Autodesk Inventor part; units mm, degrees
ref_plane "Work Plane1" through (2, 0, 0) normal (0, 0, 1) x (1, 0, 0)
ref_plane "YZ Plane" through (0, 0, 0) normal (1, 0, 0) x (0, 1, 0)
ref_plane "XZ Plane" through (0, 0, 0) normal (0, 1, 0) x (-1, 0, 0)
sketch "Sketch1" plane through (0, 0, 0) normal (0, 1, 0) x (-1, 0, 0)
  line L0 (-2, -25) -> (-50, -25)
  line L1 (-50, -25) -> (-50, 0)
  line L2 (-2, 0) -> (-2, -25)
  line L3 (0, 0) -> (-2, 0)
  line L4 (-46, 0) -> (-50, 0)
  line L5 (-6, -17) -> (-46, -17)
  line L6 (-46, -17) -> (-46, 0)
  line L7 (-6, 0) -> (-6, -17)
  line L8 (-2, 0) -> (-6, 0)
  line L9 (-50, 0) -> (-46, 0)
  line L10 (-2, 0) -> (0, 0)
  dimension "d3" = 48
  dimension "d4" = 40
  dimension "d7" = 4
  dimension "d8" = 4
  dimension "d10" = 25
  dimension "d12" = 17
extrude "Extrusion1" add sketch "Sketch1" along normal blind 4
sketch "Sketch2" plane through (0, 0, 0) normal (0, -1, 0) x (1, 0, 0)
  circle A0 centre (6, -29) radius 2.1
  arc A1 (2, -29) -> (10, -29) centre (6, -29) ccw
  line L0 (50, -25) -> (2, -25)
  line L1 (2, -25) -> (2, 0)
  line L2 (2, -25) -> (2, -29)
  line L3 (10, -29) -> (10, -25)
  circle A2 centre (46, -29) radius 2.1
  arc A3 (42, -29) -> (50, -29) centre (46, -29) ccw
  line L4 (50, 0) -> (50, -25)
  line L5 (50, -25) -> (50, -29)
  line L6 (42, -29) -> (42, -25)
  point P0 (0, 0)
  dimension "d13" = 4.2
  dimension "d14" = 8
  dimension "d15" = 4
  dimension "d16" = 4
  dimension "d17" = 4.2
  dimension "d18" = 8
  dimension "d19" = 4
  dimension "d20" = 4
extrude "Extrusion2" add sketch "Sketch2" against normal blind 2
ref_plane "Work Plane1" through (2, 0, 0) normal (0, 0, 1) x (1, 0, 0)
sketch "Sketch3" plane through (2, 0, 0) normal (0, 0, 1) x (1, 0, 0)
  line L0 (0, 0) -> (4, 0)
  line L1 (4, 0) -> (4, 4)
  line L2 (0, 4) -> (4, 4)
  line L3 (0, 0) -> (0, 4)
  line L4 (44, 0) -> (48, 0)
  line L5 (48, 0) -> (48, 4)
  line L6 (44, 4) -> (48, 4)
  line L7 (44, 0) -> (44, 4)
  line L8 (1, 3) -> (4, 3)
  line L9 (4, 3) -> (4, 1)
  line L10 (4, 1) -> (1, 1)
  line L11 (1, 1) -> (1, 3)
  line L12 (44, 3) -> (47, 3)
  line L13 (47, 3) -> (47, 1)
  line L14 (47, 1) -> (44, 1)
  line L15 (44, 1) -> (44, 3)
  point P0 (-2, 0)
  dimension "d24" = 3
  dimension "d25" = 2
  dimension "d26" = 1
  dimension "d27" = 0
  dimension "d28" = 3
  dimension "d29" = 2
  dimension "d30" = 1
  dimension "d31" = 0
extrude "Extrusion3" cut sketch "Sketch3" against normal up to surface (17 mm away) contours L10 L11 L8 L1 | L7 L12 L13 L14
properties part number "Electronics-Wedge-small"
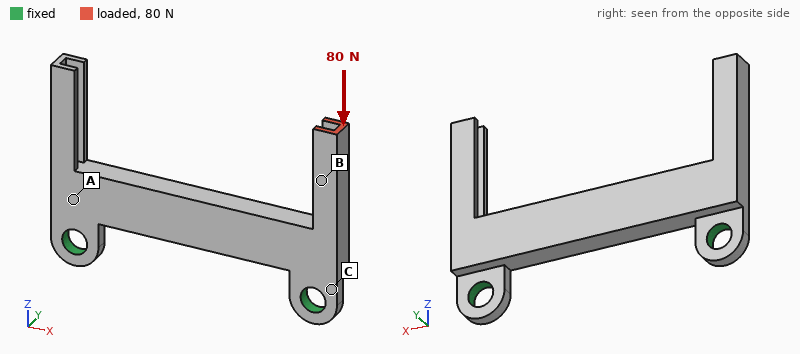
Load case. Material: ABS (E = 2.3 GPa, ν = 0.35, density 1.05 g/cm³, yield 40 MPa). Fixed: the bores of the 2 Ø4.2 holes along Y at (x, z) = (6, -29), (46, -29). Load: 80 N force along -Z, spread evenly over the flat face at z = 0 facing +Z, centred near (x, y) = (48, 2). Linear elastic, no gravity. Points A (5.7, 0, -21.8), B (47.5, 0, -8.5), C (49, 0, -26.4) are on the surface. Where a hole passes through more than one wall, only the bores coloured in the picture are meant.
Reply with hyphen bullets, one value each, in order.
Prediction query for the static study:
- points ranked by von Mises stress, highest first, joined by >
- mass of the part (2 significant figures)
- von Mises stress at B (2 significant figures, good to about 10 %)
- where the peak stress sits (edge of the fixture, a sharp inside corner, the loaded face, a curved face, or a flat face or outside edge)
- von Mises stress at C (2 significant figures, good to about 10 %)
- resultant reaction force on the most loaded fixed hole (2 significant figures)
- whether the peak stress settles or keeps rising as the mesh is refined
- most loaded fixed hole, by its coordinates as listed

- B > C > A
- 2.2 g
- 8.0 MPa
- edge of the fixture
- 3.1 MPa
- 83 N
- keeps rising
- (46, -29)
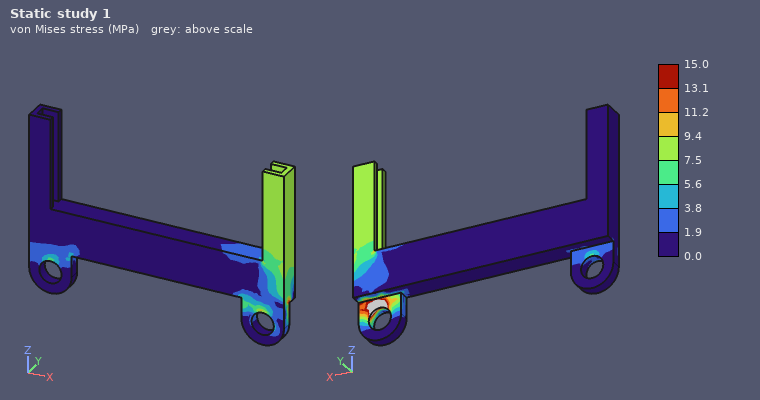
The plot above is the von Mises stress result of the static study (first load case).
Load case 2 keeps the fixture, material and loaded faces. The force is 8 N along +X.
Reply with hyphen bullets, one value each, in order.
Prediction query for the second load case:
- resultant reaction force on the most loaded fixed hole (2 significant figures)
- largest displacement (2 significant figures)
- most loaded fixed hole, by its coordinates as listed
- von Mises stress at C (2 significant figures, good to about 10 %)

- 11 N
- 0.62 mm
- (6, -29)
- 1.6 MPa
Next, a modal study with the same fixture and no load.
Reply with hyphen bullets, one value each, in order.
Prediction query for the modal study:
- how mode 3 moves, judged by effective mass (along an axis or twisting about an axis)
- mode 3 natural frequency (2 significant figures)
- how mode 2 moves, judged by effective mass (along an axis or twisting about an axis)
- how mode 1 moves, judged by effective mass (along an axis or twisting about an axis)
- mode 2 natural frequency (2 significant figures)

- along Y
- 2200 Hz
- twisting about Z
- along Y
- 1400 Hz
